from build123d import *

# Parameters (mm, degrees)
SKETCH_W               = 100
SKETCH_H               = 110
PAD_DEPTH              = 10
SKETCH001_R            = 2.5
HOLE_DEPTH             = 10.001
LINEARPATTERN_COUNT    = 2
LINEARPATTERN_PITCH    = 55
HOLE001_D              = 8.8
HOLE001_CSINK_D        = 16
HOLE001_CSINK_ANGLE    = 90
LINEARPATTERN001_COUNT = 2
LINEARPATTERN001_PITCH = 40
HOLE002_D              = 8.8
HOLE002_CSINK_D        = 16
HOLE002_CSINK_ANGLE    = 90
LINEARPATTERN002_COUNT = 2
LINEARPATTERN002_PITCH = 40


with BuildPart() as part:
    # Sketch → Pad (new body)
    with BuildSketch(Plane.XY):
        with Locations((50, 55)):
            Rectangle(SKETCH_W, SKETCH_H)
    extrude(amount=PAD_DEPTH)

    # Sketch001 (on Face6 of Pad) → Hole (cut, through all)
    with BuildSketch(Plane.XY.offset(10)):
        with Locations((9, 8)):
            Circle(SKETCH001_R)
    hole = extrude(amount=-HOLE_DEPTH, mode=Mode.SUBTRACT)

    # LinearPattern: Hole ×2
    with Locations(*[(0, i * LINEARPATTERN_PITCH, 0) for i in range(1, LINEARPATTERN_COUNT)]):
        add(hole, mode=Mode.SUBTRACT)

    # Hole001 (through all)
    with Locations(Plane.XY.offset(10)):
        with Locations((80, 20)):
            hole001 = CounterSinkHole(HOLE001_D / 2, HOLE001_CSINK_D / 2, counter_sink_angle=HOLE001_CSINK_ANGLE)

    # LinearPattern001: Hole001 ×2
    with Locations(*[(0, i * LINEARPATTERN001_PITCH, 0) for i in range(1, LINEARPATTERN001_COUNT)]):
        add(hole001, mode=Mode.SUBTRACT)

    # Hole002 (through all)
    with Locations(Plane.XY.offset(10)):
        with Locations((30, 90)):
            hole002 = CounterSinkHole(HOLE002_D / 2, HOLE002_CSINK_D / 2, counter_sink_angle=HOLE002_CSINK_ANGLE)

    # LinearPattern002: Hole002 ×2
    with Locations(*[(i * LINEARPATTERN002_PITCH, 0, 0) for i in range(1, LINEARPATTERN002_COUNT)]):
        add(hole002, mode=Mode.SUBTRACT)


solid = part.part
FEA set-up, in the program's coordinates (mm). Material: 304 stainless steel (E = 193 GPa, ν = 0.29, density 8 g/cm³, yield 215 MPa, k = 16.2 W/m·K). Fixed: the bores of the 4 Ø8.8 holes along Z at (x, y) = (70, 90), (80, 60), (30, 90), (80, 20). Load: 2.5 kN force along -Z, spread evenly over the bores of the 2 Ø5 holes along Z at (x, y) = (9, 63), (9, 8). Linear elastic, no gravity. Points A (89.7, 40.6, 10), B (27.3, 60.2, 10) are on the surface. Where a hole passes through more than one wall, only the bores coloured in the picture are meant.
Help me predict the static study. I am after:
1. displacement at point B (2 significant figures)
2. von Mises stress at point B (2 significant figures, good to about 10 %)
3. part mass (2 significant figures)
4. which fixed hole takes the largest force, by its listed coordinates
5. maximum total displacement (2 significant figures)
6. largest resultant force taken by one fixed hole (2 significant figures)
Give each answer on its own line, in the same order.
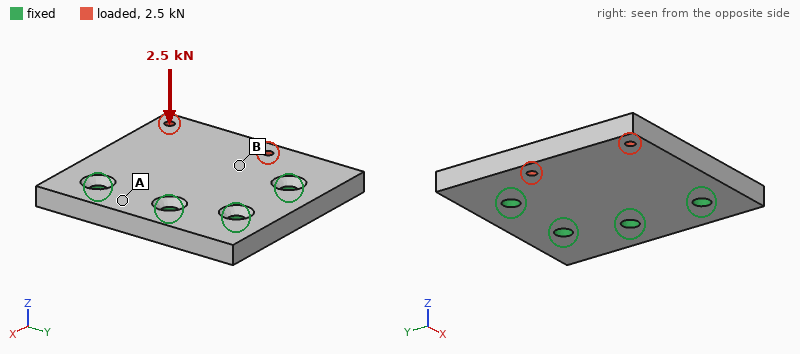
0.031 mm
41 MPa
850 g
(30, 90)
0.18 mm
2.4 kN
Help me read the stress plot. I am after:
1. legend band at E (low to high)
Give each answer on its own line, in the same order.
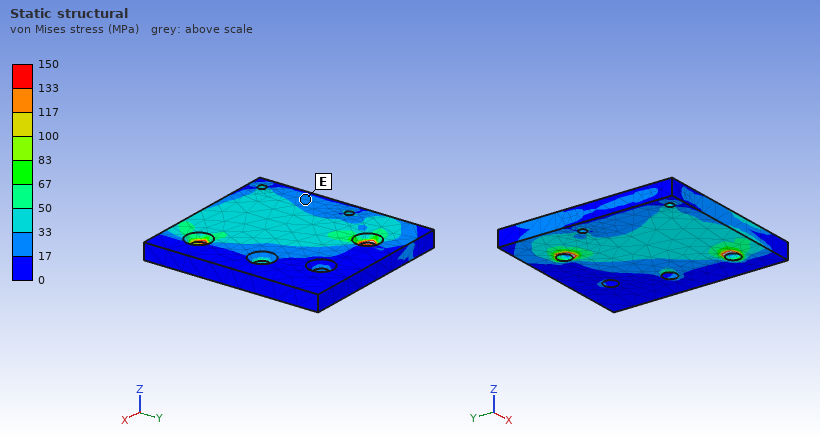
17 to 33 MPa
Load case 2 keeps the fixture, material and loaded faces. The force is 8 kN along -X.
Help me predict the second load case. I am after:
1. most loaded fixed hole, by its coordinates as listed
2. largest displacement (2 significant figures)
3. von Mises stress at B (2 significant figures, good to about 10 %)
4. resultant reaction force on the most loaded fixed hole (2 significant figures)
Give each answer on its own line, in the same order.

(80, 20)
8.8 µm
12 MPa
4.5 kN
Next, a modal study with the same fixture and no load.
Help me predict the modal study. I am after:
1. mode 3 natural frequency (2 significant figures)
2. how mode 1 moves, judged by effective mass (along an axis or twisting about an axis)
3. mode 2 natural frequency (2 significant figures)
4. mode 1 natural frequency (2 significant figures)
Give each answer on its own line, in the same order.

7500 Hz
along Z
5500 Hz
1900 Hz
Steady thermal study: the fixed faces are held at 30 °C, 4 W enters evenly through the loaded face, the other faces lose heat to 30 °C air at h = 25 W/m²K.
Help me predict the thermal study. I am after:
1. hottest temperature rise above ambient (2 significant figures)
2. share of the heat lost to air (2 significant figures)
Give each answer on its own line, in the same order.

15 K
46 %
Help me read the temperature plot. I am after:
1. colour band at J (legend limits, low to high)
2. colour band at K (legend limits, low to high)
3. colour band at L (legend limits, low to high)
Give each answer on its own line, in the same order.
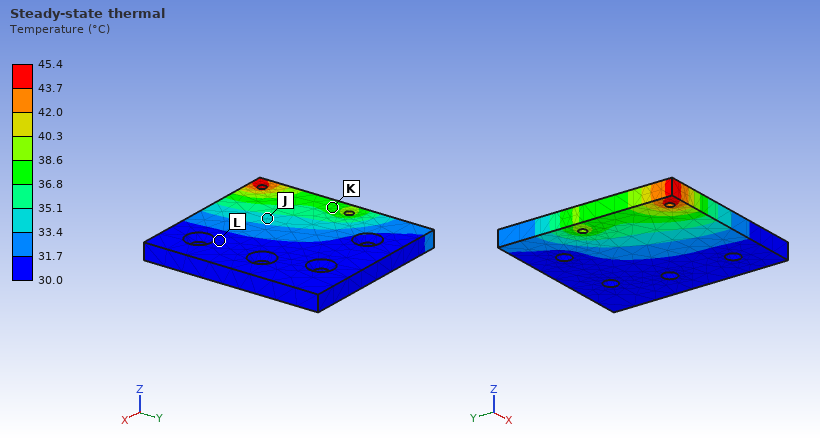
33.4 to 35.1 °C
36.8 to 38.6 °C
30.0 to 31.7 °C
